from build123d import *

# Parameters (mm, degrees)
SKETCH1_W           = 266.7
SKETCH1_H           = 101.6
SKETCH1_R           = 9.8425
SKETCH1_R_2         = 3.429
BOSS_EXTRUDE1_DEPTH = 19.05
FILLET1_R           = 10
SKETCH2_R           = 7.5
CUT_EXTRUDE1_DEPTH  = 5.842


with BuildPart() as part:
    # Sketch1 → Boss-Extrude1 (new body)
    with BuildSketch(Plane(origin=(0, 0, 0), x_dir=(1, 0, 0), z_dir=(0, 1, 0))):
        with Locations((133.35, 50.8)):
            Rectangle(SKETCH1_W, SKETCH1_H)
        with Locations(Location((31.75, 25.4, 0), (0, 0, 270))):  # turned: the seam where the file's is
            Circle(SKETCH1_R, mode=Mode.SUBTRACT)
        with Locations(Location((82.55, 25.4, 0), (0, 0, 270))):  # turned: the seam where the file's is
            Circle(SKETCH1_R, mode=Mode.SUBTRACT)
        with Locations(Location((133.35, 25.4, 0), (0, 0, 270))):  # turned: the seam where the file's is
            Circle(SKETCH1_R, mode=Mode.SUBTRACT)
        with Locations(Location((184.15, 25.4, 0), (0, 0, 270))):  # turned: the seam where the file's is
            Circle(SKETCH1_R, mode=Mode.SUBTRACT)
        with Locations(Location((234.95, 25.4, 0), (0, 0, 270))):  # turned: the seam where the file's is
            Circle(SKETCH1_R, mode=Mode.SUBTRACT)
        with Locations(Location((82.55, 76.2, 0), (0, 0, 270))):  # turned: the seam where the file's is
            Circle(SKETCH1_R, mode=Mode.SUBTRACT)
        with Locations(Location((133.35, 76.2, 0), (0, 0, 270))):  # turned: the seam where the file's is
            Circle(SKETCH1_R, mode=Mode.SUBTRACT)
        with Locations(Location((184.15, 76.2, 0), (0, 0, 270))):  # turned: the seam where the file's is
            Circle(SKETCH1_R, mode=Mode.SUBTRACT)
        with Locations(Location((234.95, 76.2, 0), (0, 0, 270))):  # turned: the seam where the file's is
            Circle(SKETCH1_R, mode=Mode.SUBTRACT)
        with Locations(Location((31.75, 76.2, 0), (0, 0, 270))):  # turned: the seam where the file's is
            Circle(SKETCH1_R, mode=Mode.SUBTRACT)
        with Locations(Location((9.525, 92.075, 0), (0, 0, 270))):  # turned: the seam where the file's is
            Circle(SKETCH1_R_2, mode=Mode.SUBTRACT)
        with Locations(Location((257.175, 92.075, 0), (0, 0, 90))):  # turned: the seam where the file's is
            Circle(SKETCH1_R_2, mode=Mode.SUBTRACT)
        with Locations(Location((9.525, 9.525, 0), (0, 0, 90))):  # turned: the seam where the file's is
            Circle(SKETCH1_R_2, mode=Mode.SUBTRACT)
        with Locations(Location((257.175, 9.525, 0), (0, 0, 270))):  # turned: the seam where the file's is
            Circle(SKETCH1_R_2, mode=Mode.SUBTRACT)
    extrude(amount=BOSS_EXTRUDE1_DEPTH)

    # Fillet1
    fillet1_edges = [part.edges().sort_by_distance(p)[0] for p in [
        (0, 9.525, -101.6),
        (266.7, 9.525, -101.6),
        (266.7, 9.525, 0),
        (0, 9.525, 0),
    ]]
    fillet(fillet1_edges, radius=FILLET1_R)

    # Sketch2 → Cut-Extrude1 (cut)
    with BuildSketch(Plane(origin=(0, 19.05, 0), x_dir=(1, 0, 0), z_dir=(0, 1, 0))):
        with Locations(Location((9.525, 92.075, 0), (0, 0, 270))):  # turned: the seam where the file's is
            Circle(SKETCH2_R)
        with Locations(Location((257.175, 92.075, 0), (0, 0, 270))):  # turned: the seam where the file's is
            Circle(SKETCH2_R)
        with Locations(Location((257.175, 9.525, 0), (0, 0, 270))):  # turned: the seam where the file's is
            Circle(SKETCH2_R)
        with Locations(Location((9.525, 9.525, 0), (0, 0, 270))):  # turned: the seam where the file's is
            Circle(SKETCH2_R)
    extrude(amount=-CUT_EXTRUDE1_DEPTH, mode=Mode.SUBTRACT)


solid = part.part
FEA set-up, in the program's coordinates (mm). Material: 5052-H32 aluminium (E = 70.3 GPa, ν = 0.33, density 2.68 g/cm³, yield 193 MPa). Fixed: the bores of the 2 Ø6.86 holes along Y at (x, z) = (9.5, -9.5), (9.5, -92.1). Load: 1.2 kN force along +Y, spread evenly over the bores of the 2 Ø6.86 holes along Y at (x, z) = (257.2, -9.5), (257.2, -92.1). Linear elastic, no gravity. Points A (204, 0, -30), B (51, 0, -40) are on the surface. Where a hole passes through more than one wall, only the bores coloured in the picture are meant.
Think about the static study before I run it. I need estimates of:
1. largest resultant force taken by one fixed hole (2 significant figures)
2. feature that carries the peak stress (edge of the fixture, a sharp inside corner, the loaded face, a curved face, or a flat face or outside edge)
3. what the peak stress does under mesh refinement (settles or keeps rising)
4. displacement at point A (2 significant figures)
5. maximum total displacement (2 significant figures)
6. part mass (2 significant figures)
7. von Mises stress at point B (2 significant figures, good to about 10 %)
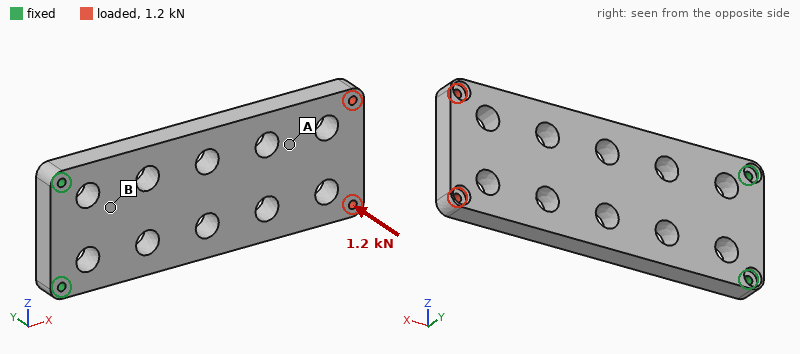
610 N
edge of the fixture
keeps rising
1.9 mm
2.8 mm
1.2 kg
45 MPa
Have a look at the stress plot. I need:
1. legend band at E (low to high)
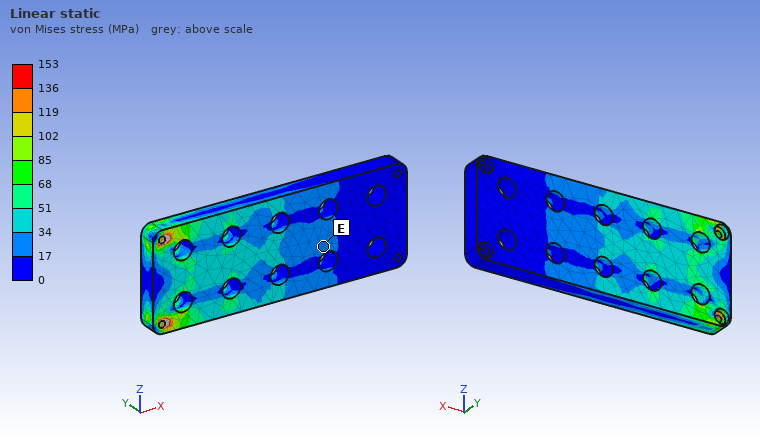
17 to 34 MPa
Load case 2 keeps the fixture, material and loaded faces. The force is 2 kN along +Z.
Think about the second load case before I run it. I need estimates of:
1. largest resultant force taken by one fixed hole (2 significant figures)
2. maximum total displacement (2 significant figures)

5.9 kN
0.16 mm
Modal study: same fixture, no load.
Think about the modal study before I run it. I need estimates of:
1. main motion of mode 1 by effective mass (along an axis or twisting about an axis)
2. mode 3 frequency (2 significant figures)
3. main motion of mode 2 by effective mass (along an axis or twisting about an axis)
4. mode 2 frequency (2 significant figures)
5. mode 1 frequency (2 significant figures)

along Y
1100 Hz
along Z
1000 Hz
180 Hz
